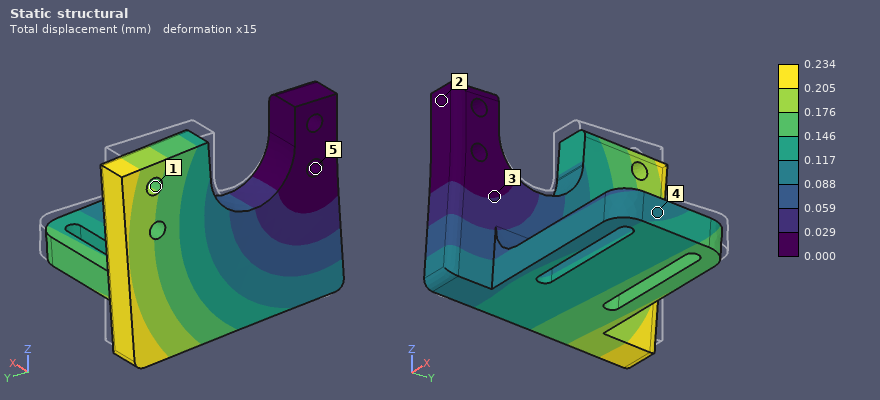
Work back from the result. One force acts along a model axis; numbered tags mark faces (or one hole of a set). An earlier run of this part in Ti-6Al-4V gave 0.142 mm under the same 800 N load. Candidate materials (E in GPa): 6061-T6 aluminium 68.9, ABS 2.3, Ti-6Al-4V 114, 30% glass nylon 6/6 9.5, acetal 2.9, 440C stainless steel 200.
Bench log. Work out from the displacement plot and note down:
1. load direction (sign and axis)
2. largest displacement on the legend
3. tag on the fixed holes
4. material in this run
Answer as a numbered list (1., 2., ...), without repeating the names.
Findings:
1. -Z
2. 0.234 mm
3. 5
4. 6061-T6 aluminium
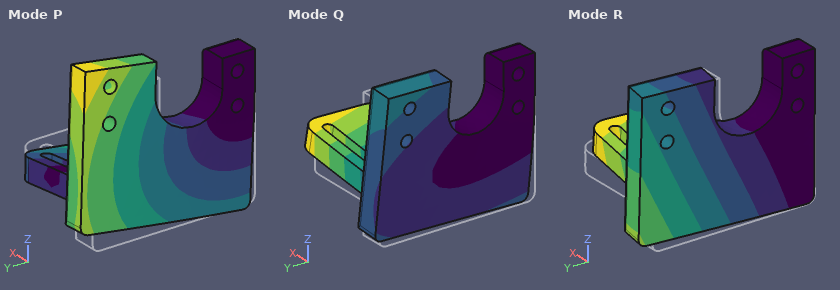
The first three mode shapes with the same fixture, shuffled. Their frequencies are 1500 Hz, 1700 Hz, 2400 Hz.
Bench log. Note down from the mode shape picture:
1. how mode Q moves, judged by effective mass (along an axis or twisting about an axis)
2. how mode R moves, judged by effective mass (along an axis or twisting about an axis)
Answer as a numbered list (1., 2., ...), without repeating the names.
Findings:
1. along Z
2. along X
